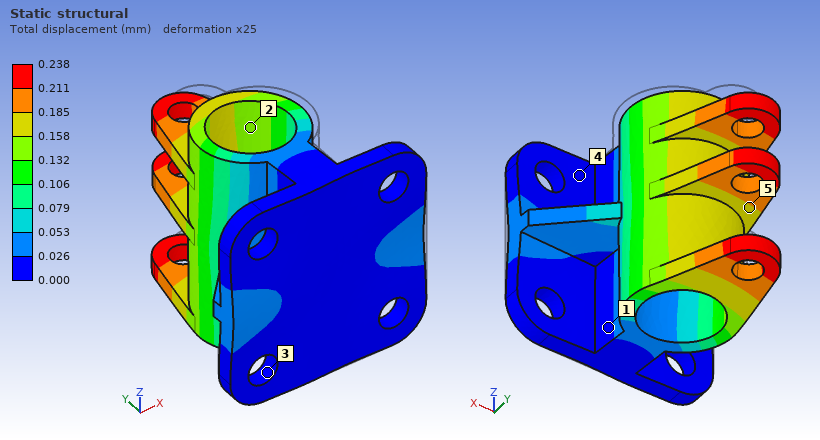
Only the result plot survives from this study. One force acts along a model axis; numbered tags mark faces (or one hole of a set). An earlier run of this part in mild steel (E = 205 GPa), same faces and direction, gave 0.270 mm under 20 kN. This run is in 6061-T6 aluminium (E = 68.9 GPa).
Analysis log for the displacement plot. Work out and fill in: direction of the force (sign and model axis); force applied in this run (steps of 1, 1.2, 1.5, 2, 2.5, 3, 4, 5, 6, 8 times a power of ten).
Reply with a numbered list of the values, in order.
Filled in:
1. -X
2. 6 kN
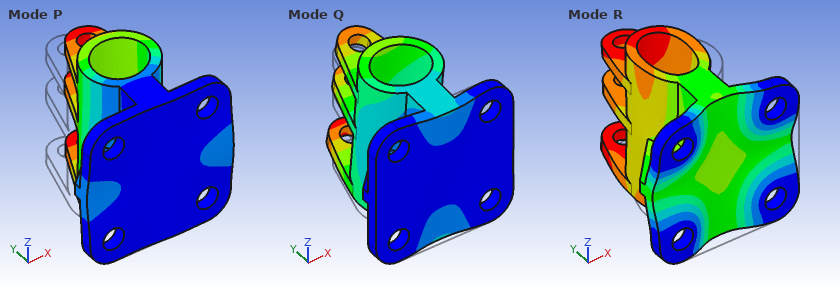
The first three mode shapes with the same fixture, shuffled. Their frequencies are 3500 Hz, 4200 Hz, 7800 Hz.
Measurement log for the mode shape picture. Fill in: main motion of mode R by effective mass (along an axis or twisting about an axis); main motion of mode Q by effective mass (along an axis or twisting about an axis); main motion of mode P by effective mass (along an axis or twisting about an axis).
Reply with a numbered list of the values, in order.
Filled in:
1. along Y
2. along Z
3. along X
